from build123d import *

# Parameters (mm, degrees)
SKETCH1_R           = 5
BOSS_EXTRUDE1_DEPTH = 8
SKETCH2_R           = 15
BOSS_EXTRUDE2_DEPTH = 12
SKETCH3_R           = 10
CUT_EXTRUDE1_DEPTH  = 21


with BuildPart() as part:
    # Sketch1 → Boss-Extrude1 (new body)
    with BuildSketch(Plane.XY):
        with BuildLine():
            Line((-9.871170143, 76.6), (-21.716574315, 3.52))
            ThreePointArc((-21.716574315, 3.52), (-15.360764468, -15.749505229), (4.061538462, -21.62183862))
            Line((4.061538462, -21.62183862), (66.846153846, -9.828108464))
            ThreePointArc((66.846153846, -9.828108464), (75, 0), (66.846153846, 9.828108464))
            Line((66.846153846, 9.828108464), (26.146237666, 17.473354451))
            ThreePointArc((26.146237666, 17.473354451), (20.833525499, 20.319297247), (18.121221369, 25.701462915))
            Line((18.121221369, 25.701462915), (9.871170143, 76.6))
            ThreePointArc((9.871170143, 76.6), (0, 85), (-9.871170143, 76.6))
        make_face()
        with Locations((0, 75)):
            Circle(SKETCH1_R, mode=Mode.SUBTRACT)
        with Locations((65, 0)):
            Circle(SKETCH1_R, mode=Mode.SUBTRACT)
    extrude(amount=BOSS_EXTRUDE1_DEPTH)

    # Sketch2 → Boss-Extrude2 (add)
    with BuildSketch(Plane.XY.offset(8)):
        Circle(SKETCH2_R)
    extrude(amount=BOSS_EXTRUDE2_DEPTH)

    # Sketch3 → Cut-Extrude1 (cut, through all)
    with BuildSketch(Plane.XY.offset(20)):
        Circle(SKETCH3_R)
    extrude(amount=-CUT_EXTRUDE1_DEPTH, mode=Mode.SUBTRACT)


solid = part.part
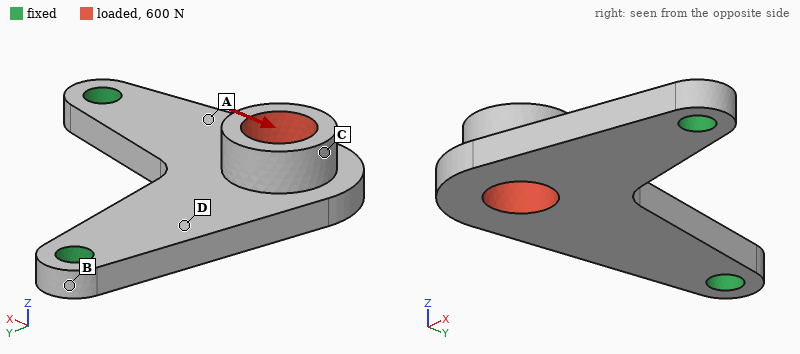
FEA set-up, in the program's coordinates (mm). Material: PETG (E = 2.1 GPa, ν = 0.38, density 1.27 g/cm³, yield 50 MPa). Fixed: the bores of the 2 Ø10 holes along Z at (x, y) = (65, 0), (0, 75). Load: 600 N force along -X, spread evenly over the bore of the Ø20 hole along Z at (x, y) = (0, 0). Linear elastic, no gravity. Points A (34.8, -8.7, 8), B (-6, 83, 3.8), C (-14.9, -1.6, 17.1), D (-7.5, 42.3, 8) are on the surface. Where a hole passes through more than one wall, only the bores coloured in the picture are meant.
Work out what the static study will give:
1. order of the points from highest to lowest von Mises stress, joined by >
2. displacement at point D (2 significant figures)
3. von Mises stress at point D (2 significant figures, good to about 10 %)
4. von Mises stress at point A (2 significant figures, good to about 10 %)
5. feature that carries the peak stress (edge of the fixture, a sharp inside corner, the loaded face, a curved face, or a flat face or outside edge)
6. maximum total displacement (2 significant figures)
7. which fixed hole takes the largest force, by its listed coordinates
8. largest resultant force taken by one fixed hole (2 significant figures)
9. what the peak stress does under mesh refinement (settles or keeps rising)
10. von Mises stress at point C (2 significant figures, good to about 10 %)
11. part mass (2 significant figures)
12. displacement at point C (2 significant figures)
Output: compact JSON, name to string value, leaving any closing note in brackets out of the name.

{"order of the points from highest to lowest von Mises stress, joined by >": "A > D > C > B", "displacement at point D": "0.34 mm", "von Mises stress at point D": "4.4 MPa", "von Mises stress at point A": "6.8 MPa", "feature that carries the peak stress": "edge of the fixture", "maximum total displacement": "1.4 mm", "which fixed hole takes the largest force, by its listed coordinates": "(65, 0)", "largest resultant force taken by one fixed hole": "580 N", "what the peak stress does under mesh refinement": "keeps rising", "von Mises stress at point C": "2.6 MPa", "part mass": "50 g", "displacement at point C": "1.3 mm"}
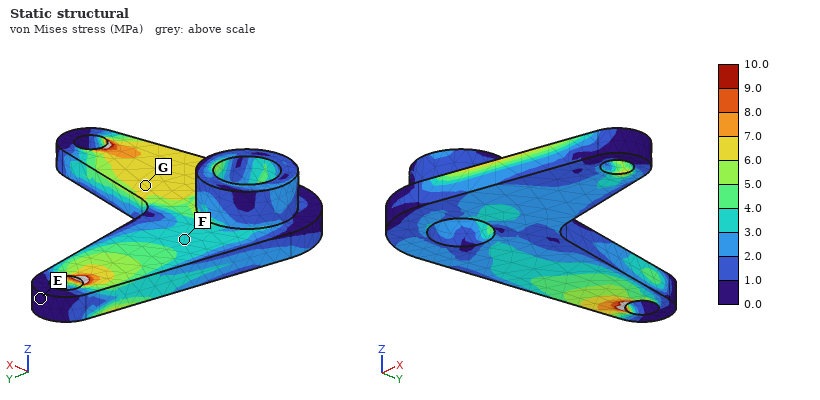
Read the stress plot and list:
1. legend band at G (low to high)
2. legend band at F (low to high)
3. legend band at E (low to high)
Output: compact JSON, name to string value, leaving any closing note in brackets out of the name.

{"legend band at G": "6.0 to 7.0 MPa", "legend band at F": "3.0 to 4.0 MPa", "legend band at E": "0.0 to 1.0 MPa"}
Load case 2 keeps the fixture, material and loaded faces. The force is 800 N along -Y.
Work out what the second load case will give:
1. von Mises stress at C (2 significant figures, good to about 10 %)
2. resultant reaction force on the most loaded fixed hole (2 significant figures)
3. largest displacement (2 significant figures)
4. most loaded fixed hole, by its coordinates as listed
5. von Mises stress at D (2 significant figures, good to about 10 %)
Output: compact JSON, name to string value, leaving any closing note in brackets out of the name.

{"von Mises stress at C": "1.9 MPa", "resultant reaction force on the most loaded fixed hole": "750 N", "largest displacement": "1.6 mm", "most loaded fixed hole, by its coordinates as listed": "(0, 75)", "von Mises stress at D": "7.5 MPa"}
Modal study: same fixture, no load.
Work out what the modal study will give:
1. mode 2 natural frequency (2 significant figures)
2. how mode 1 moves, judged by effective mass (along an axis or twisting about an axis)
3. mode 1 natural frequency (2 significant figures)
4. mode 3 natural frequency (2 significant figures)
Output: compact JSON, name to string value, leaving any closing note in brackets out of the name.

{"mode 2 natural frequency": "1100 Hz", "how mode 1 moves, judged by effective mass": "along Z", "mode 1 natural frequency": "310 Hz", "mode 3 natural frequency": "1300 Hz"}
